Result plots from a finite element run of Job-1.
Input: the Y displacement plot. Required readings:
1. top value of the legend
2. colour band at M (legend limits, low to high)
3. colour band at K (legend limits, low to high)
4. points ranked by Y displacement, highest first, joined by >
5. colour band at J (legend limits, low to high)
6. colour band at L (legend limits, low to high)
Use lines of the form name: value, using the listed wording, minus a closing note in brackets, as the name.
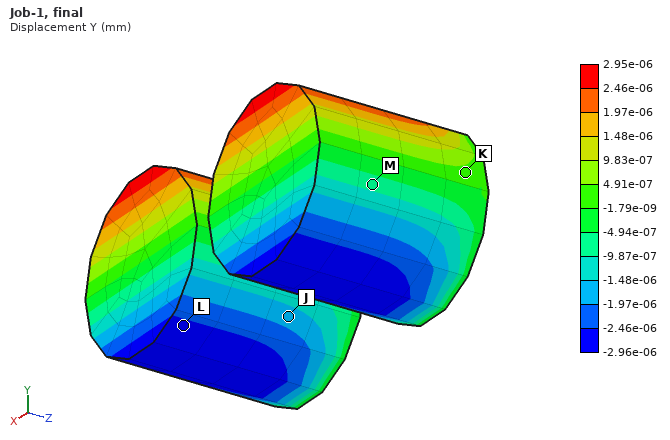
top value of the legend: 2.95e-06 mm
colour band at M: -9.87e-07 to -4.94e-07 mm
colour band at K: -1.79e-09 to 4.91e-07 mm
points ranked by Y displacement, highest first, joined by >: K > M > J > L
colour band at J: -1.97e-06 to -1.48e-06 mm
colour band at L: -2.96e-06 to -2.46e-06 mm
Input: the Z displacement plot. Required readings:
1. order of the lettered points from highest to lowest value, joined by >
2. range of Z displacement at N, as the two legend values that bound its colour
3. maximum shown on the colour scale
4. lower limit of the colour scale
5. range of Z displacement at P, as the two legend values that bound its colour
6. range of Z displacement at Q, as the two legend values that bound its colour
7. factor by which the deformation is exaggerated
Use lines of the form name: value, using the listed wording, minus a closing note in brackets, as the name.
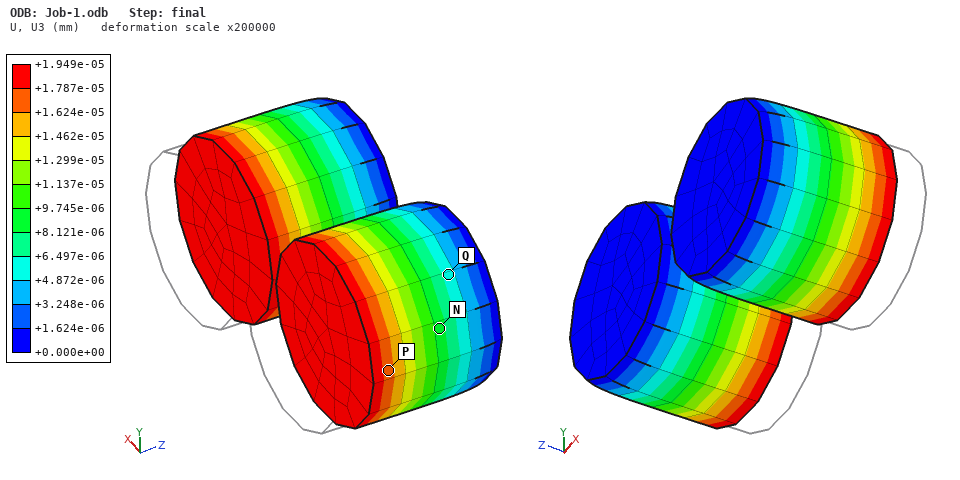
order of the lettered points from highest to lowest value, joined by >: P > N > Q
range of Z displacement at N, as the two legend values that bound its colour: +8.121e-06 to +9.745e-06 mm
maximum shown on the colour scale: +1.949e-05 mm
lower limit of the colour scale: +0.000e+00 mm
range of Z displacement at P, as the two legend values that bound its colour: +1.624e-05 to +1.787e-05 mm
range of Z displacement at Q, as the two legend values that bound its colour: +4.872e-06 to +6.497e-06 mm
factor by which the deformation is exaggerated: 200000
